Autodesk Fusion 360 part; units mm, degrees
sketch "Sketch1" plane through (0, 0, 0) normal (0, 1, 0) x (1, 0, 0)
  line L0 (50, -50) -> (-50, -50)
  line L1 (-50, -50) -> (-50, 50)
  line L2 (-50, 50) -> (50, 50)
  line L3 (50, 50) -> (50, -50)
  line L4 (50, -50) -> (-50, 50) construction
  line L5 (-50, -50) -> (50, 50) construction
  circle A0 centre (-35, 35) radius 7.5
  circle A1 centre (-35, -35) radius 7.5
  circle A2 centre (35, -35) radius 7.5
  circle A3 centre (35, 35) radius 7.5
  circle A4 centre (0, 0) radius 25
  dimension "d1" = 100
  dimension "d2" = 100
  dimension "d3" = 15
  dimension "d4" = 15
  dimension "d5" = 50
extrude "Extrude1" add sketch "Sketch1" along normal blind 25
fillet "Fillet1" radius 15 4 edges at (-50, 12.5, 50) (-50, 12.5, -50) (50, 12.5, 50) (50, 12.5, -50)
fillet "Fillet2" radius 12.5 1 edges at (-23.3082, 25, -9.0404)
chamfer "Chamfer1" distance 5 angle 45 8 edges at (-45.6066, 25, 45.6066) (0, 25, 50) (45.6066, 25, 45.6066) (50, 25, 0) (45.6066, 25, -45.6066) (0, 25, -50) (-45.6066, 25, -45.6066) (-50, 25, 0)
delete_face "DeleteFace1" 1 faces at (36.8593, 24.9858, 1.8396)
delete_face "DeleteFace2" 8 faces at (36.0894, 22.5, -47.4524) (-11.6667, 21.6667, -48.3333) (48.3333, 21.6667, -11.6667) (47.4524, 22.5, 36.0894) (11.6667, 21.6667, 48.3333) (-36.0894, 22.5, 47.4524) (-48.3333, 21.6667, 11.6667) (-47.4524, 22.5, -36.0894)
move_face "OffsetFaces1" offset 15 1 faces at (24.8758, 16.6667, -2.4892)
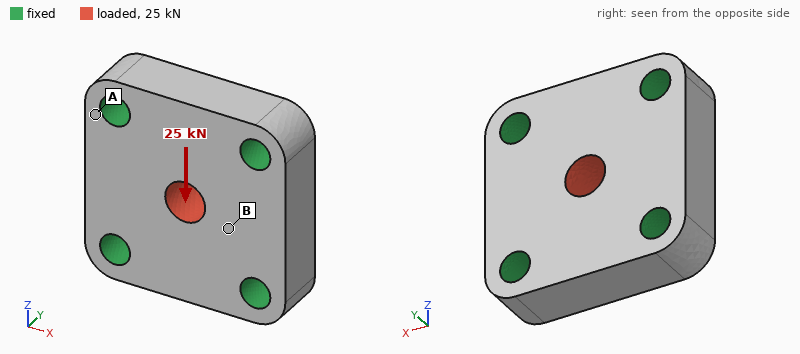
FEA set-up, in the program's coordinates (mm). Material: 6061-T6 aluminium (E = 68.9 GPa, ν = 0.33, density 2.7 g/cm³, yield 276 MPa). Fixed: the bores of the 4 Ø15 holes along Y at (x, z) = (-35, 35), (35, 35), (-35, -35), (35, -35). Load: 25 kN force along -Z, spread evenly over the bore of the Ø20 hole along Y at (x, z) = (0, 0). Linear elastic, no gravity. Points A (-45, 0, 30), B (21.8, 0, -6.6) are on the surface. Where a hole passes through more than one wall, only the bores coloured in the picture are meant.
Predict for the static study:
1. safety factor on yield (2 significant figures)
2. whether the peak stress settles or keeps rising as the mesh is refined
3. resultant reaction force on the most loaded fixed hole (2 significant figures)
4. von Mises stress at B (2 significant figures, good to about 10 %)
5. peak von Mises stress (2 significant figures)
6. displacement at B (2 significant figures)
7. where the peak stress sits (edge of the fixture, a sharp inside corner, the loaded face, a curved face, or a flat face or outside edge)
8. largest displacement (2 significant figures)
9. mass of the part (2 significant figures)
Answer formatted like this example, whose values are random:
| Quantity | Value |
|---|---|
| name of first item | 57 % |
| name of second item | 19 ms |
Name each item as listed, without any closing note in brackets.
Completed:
| Quantity | Value |
|---|---|
| safety factor on yield | 9.9 |
| whether the peak stress settles or keeps rising as the mesh is refined | settles |
| resultant reaction force on the most loaded fixed hole | 7.0 kN |
| von Mises stress at B | 8.3 MPa |
| peak von Mises stress | 28 MPa |
| displacement at B | 3.1 µm |
| where the peak stress sits | the loaded face |
| largest displacement | 8.2 µm |
| mass of the part | 590 g |
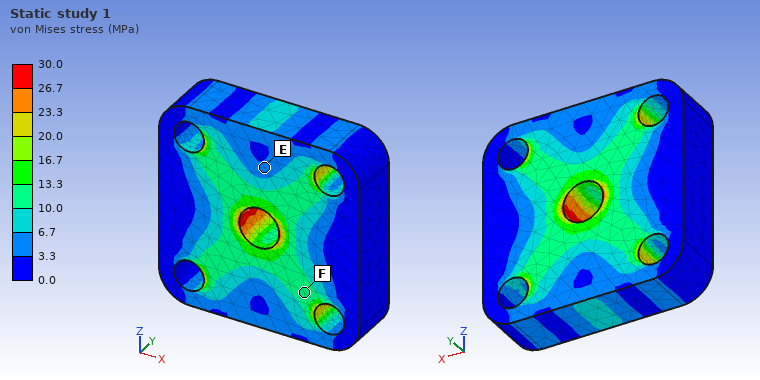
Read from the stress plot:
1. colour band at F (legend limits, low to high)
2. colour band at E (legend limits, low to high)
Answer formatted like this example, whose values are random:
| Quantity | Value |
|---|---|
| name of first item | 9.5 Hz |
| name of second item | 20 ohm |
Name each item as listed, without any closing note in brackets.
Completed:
| Quantity | Value |
|---|---|
| colour band at F | 10.0 to 13.3 MPa |
| colour band at E | 3.3 to 6.7 MPa |
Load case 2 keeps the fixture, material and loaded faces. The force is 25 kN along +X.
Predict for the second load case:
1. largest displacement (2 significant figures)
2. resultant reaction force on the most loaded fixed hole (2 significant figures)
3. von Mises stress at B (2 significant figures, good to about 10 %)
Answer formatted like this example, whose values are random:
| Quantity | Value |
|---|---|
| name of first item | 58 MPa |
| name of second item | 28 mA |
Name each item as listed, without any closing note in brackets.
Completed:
| Quantity | Value |
|---|---|
| largest displacement | 8.2 µm |
| resultant reaction force on the most loaded fixed hole | 7.0 kN |
| von Mises stress at B | 9.7 MPa |
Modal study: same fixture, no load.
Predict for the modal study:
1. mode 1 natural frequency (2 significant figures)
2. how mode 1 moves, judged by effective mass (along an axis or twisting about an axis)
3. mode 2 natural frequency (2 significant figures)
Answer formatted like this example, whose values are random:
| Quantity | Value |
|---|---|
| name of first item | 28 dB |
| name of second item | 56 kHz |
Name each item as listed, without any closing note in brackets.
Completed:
| Quantity | Value |
|---|---|
| mode 1 natural frequency | 15 kHz |
| how mode 1 moves, judged by effective mass | along Y |
| mode 2 natural frequency | 20 kHz |
